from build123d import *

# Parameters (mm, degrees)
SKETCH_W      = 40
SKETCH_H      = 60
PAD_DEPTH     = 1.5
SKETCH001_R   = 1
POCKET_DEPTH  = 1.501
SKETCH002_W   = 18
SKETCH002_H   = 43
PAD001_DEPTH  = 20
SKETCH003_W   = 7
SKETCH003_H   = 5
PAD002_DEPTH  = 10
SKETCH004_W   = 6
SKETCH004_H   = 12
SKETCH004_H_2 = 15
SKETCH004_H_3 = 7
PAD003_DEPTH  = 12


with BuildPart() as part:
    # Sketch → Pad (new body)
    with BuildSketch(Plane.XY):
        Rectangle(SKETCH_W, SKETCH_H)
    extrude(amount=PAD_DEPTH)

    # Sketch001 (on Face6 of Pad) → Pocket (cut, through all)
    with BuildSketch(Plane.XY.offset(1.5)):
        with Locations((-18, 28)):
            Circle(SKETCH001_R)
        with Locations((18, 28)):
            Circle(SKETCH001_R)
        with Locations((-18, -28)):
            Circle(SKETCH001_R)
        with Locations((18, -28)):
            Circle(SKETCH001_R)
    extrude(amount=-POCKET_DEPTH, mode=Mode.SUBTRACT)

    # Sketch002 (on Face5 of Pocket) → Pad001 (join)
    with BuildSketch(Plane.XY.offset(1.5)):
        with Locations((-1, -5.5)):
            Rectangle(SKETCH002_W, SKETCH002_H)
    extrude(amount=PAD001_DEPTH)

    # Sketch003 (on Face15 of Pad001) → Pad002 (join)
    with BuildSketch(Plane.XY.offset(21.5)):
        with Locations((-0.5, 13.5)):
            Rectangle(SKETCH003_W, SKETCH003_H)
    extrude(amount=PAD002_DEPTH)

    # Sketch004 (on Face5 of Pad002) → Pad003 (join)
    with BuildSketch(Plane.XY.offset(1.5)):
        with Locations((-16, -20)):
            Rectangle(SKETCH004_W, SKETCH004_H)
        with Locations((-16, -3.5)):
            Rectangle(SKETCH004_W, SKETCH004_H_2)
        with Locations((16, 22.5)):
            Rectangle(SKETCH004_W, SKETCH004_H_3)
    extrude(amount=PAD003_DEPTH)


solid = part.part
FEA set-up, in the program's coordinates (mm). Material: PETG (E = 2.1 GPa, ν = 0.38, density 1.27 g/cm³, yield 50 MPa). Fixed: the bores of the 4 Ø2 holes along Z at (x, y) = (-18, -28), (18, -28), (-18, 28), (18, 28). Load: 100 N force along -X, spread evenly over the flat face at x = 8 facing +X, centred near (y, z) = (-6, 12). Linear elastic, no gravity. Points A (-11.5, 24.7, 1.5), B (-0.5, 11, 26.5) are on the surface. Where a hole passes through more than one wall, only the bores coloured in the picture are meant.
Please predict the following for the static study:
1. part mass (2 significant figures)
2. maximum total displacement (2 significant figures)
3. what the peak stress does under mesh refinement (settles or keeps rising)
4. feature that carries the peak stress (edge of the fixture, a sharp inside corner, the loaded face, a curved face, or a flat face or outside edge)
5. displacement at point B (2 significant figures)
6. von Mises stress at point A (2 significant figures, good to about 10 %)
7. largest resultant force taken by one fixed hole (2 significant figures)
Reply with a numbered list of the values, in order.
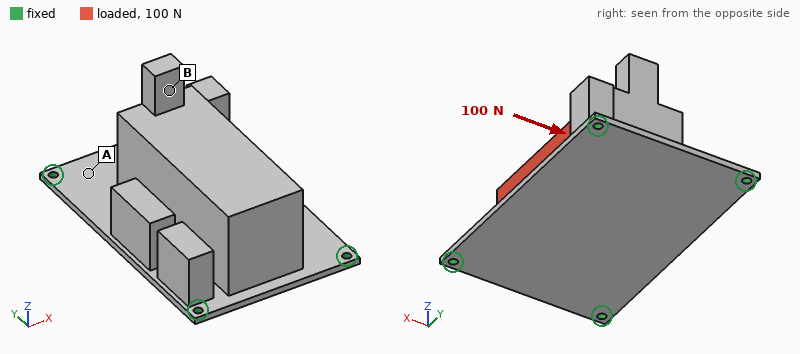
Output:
1. 28 g
2. 0.79 mm
3. keeps rising
4. edge of the fixture
5. 0.66 mm
6. 4.9 MPa
7. 47 N
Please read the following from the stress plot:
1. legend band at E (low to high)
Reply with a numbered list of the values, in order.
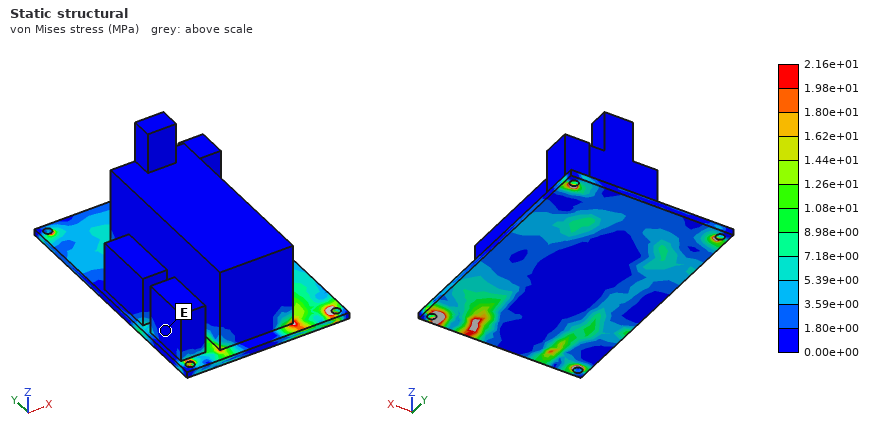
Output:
1. 0.00e+00 to 1.80e+00 MPa
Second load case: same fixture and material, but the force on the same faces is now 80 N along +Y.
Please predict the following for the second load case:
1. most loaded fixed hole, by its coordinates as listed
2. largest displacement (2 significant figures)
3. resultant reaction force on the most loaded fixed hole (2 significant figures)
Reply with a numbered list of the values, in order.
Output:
1. (-18, -28)
2. 0.43 mm
3. 29 N
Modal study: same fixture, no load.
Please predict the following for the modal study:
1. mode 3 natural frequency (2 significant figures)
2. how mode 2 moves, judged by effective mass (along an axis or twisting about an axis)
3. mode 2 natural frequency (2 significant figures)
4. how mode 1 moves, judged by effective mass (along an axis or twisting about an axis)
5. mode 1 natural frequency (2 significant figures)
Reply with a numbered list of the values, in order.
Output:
1. 700 Hz
2. along X
3. 480 Hz
4. along Z
5. 370 Hz
